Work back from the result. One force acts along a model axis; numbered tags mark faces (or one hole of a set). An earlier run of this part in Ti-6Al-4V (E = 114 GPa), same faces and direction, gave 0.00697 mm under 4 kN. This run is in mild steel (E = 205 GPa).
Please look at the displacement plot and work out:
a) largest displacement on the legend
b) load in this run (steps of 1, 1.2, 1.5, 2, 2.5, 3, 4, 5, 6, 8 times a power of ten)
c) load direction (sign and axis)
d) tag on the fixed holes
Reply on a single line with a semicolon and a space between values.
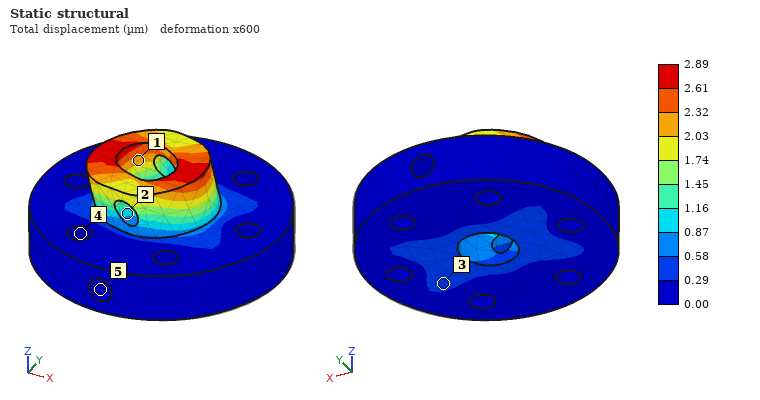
2.89 µm; 3 kN; -X; 4
